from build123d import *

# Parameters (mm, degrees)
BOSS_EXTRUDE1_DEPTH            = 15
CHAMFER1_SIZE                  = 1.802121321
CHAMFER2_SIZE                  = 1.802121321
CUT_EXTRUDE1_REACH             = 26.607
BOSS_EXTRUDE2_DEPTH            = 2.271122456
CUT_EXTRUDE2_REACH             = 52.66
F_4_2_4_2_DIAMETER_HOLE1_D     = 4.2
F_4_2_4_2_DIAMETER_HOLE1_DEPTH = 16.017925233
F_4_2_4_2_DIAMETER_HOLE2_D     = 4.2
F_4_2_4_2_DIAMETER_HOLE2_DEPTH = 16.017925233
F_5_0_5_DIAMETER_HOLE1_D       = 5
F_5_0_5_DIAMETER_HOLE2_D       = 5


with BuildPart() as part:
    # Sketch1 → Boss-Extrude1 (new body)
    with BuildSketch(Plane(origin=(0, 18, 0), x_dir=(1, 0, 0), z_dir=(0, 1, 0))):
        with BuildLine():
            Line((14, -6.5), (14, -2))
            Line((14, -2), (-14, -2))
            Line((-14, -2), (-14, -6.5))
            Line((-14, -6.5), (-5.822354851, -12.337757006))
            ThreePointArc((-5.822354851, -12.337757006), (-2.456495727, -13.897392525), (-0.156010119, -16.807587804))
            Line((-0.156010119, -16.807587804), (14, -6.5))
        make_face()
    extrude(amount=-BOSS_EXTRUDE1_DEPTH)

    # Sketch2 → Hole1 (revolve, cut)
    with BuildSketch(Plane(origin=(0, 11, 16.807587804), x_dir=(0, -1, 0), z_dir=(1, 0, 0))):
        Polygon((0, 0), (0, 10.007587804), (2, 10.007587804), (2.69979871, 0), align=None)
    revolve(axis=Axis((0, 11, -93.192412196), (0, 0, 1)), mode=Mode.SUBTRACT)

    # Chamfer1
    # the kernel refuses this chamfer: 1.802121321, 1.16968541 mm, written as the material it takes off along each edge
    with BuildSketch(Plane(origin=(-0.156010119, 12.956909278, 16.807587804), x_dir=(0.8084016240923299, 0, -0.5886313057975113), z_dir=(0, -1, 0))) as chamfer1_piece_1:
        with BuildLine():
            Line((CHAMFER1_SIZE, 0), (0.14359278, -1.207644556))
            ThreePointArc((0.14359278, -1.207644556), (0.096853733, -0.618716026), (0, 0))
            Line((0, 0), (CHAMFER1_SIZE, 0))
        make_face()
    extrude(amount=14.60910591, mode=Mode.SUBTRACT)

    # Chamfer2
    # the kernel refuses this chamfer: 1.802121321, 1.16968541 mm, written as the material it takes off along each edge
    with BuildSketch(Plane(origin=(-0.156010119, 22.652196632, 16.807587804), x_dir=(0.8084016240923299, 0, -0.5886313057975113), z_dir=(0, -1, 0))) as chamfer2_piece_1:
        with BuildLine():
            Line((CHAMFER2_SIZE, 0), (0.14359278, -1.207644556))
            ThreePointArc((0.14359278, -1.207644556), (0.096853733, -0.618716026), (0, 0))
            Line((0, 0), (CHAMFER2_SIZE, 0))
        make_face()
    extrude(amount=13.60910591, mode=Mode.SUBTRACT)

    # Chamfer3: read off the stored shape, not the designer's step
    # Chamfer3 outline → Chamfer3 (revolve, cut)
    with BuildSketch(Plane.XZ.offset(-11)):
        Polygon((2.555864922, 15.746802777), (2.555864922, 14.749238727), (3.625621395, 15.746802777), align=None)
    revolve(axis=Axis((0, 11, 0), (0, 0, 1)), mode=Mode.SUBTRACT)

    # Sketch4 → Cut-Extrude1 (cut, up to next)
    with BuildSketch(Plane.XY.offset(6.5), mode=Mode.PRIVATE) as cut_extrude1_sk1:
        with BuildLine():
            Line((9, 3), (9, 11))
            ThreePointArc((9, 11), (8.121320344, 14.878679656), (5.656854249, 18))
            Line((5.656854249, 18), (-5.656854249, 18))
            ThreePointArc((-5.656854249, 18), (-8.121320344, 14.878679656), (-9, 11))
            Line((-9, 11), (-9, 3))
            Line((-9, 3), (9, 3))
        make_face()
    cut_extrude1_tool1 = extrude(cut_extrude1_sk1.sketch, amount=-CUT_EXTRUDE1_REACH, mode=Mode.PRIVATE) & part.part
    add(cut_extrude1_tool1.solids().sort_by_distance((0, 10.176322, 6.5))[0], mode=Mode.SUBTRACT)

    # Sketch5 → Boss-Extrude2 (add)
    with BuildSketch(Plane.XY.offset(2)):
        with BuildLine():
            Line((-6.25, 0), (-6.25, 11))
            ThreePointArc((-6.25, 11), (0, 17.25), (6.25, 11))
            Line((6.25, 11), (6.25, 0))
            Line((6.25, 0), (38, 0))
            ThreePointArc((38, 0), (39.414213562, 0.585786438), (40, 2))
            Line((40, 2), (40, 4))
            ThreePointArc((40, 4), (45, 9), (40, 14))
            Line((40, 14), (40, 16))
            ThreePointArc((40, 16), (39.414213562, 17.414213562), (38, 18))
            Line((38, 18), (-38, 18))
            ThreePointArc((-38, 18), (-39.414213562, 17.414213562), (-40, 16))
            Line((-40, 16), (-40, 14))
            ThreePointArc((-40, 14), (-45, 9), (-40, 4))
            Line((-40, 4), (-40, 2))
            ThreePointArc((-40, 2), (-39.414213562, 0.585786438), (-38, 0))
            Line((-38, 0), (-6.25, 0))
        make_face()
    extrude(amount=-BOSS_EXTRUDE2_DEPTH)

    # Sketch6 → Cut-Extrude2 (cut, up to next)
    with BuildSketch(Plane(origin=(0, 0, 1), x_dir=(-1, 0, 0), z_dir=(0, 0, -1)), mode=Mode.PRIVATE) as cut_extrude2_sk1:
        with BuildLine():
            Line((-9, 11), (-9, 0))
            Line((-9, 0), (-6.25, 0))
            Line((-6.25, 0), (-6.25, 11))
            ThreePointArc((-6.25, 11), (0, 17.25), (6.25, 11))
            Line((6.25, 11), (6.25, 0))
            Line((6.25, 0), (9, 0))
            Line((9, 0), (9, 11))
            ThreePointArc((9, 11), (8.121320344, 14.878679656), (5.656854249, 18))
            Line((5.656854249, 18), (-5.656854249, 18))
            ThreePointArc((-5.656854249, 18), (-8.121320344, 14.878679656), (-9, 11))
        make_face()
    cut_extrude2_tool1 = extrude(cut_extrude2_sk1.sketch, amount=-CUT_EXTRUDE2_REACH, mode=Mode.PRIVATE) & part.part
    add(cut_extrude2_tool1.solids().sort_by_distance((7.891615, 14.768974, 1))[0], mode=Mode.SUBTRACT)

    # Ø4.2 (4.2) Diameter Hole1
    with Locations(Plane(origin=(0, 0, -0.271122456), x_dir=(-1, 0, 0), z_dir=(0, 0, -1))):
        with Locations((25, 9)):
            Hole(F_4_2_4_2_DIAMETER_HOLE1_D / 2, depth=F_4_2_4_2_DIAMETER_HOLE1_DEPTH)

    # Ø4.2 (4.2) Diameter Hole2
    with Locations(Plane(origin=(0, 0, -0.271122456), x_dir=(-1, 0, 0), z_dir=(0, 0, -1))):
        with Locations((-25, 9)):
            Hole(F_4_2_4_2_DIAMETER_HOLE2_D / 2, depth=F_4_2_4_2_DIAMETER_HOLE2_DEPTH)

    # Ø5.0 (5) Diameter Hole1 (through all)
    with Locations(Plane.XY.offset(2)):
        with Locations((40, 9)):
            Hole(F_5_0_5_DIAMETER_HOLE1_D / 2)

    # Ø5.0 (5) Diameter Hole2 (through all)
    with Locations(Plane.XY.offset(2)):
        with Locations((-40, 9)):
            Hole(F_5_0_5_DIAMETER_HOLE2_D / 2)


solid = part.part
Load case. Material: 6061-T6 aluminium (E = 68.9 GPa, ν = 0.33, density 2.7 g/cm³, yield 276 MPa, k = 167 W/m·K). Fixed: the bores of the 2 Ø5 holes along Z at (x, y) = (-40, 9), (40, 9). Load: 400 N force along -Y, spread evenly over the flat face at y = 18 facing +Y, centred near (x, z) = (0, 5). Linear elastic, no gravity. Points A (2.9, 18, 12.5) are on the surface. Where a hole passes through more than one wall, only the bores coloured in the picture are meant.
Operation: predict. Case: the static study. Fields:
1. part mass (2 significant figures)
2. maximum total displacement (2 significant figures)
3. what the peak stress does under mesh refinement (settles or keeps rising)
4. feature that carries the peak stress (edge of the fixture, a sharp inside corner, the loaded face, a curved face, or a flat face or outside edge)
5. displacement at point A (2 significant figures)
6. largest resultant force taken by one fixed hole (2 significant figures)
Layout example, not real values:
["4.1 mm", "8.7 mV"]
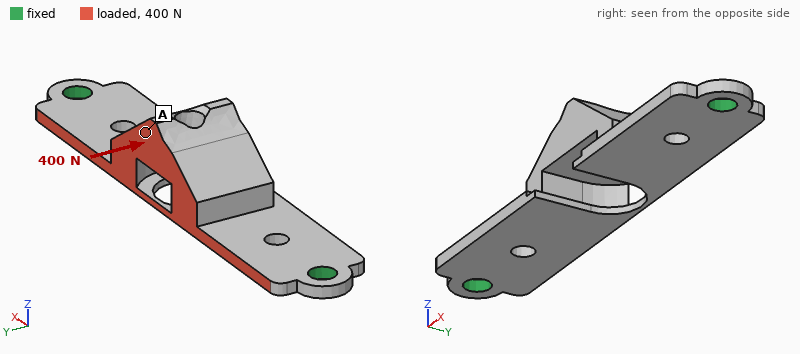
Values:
["15 g", "0.23 mm", "keeps rising", "edge of the fixture", "0.20 mm", "230 N"]
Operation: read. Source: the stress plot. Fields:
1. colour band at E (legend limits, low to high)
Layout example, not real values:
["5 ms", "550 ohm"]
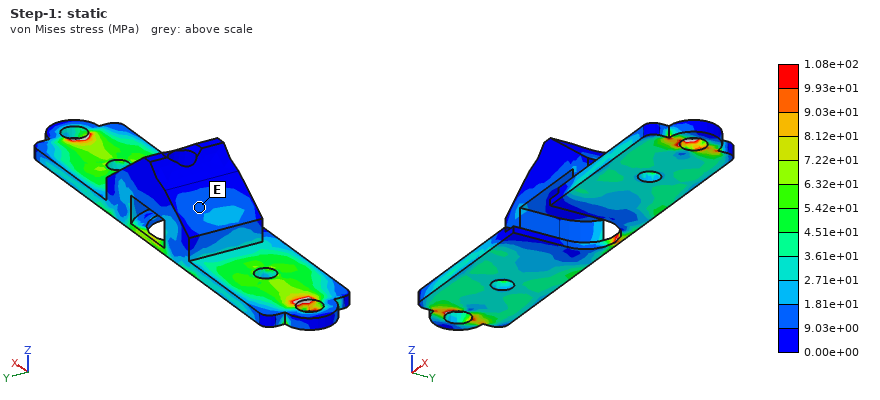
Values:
["9.03e+00 to 1.81e+01 MPa"]
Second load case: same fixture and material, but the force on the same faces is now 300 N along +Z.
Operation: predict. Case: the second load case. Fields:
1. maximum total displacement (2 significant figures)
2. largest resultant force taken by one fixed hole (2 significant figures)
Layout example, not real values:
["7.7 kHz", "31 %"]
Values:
["0.39 mm", "250 N"]
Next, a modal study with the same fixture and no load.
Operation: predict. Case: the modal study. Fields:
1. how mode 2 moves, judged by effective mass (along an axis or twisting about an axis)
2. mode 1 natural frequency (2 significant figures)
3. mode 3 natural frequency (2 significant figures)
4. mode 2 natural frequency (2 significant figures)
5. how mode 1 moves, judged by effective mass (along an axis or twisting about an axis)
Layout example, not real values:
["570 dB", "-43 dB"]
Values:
["along Y", "1900 Hz", "4100 Hz", "2200 Hz", "along Z"]
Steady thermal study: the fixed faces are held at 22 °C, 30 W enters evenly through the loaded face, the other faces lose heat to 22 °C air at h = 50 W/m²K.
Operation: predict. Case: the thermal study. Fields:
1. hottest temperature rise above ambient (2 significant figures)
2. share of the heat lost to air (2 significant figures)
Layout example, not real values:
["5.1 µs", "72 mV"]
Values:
["54 K", "22 %"]
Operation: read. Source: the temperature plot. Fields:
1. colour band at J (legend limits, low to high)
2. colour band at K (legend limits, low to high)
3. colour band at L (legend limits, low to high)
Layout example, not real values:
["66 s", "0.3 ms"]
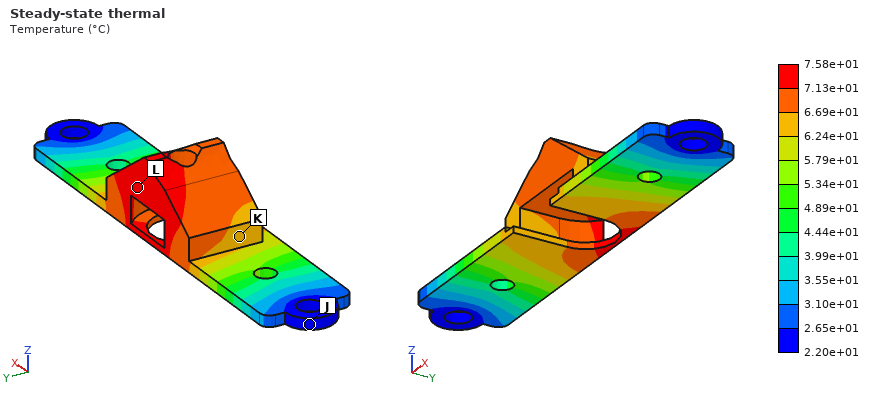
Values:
["2.20e+01 to 2.65e+01 °C", "6.24e+01 to 6.69e+01 °C", "7.13e+01 to 7.58e+01 °C"]
